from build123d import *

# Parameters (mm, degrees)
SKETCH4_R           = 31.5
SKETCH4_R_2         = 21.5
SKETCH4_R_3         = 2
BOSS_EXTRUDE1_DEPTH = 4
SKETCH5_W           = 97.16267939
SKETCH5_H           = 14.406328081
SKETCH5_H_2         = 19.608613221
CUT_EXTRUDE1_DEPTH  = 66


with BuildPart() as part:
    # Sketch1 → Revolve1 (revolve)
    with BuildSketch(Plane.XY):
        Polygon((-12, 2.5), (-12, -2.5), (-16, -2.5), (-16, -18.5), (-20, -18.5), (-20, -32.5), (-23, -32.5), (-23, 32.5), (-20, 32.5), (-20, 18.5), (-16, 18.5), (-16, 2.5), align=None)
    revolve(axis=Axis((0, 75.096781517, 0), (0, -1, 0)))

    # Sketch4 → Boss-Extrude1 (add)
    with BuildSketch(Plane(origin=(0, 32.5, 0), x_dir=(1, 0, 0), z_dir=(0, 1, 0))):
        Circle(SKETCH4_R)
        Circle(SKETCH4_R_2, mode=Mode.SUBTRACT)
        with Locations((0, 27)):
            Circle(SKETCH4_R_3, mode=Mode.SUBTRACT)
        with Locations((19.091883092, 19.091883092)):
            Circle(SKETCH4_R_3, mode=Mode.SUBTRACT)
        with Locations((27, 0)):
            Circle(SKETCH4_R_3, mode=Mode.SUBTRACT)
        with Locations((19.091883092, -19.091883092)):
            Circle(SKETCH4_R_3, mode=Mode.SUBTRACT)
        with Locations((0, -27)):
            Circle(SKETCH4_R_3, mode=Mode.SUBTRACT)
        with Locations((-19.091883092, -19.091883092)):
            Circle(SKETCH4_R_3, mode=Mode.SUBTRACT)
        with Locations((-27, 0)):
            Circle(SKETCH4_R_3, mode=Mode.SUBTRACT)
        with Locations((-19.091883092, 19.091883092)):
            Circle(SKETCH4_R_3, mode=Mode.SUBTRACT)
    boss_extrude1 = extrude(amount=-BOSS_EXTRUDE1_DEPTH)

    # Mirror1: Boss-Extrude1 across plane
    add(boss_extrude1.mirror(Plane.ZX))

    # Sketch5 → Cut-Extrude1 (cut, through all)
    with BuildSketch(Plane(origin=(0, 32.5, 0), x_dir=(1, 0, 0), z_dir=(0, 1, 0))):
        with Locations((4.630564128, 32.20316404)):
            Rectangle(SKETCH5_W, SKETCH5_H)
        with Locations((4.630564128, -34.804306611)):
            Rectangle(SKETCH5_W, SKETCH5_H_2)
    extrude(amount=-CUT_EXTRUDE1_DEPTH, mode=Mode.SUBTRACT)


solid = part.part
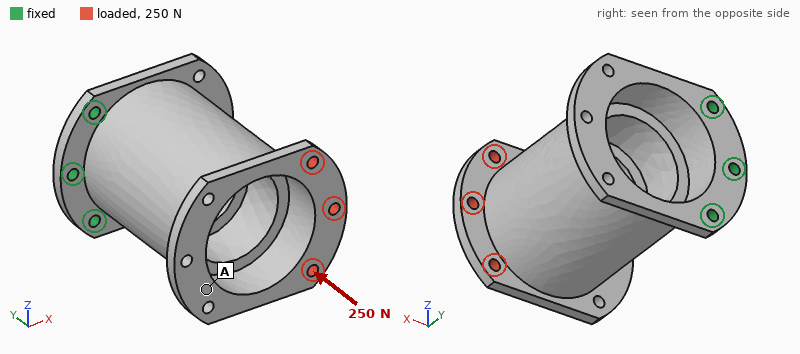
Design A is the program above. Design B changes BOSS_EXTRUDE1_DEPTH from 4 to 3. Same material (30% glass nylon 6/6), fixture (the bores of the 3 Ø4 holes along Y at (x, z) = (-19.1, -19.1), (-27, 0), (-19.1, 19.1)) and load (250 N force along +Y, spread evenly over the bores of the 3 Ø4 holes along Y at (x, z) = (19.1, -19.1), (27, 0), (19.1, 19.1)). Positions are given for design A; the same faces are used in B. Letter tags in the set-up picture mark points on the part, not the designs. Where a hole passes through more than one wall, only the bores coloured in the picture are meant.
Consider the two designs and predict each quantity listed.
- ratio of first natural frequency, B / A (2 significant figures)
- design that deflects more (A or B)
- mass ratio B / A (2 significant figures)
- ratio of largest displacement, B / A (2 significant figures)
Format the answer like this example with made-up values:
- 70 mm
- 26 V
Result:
- 0.83
- B
- 0.96
- 1.5
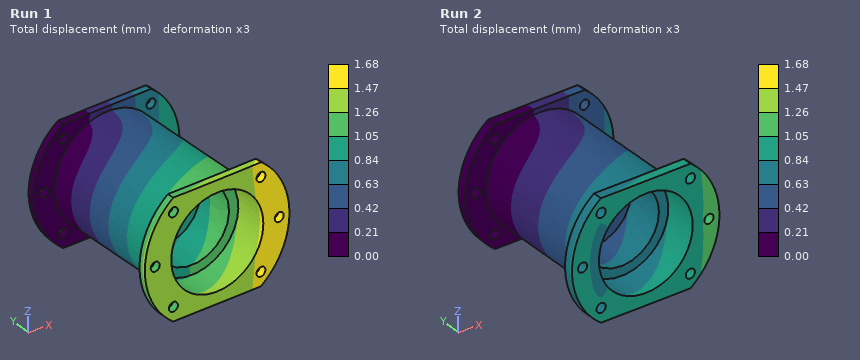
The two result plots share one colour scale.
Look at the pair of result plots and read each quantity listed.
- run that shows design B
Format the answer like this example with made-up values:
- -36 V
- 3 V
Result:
- Run 1
